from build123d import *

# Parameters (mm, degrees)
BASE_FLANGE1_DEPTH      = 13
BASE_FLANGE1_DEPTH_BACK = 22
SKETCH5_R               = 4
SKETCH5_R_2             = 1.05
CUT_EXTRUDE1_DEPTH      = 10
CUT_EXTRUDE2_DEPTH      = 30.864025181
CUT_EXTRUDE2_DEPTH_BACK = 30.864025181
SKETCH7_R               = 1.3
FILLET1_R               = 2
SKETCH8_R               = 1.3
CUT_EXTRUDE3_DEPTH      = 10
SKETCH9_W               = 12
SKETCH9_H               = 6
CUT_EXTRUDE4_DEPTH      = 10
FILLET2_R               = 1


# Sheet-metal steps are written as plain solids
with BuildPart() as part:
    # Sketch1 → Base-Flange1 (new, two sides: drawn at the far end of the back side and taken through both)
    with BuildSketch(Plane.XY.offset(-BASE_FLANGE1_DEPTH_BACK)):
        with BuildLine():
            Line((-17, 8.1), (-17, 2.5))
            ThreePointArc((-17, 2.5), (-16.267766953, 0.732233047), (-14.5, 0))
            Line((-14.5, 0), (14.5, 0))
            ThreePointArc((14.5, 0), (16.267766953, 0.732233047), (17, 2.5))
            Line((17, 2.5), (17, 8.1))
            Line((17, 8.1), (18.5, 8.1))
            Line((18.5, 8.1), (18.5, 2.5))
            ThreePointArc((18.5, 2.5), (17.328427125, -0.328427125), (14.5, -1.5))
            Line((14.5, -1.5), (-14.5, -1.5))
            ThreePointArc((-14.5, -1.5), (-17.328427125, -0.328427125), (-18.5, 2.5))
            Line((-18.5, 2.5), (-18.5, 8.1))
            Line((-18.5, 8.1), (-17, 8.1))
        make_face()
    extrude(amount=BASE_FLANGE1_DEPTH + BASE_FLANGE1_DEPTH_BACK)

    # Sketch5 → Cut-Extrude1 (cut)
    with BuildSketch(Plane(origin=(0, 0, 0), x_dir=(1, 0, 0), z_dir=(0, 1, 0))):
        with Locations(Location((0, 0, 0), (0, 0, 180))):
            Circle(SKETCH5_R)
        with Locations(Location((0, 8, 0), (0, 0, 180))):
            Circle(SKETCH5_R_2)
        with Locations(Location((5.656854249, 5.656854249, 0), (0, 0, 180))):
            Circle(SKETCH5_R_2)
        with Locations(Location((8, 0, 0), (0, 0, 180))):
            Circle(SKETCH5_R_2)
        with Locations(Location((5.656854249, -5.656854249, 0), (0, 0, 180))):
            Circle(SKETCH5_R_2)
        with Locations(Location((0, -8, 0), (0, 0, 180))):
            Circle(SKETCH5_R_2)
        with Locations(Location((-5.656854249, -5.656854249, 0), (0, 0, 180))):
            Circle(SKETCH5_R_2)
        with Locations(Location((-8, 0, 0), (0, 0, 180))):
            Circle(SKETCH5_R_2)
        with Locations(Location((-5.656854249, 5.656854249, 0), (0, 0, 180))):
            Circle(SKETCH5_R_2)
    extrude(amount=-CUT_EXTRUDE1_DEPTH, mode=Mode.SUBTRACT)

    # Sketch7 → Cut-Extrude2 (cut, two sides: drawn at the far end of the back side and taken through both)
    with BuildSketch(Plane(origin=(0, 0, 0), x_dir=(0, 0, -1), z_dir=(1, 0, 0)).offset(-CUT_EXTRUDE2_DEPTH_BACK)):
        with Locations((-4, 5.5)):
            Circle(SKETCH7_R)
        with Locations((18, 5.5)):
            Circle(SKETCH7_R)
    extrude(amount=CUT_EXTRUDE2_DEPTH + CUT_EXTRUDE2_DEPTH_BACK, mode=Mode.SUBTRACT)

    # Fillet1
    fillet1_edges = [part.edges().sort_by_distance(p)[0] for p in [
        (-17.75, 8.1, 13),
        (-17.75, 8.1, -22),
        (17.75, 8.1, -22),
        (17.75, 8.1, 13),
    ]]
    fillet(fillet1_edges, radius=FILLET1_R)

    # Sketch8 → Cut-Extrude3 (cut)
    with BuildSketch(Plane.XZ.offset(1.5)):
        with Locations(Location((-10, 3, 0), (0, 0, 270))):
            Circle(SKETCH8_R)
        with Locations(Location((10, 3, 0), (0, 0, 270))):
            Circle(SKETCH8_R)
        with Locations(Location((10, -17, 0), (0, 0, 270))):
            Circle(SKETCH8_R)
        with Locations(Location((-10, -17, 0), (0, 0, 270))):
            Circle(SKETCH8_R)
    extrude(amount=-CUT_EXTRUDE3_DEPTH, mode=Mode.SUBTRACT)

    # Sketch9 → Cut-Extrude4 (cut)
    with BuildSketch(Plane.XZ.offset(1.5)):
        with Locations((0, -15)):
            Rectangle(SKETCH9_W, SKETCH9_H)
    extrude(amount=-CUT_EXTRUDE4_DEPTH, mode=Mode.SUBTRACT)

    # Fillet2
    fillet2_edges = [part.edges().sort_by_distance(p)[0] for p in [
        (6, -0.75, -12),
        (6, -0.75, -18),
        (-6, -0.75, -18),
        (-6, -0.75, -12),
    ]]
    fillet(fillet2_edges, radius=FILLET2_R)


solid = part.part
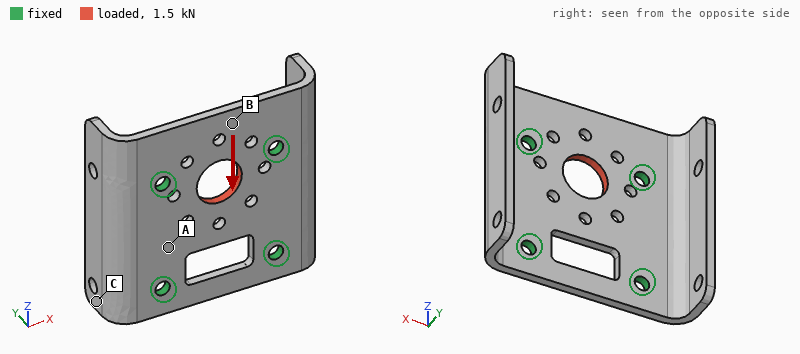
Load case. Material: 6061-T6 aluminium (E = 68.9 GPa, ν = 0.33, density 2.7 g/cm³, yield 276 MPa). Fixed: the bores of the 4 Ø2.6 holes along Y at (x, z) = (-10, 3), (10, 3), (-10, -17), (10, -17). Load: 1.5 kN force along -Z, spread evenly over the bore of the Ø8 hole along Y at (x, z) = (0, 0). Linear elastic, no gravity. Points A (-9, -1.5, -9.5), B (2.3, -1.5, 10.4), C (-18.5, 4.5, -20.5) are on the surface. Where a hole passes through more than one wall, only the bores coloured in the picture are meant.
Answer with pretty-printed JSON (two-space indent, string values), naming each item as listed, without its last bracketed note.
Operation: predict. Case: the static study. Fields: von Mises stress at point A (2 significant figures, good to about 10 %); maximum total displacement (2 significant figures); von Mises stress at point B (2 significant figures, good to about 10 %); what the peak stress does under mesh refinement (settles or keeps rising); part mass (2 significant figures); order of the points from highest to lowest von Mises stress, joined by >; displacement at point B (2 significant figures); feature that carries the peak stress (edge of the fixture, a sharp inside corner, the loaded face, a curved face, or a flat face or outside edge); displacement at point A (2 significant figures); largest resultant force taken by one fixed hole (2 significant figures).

{
  "von Mises stress at point A": "17 MPa",
  "maximum total displacement": "11 µm",
  "von Mises stress at point B": "31 MPa",
  "what the peak stress does under mesh refinement": "keeps rising",
  "part mass": "6.4 g",
  "order of the points from highest to lowest von Mises stress, joined by >": "B > A > C",
  "displacement at point B": "8.0 µm",
  "feature that carries the peak stress": "edge of the fixture",
  "displacement at point A": "2.3 µm",
  "largest resultant force taken by one fixed hole": "540 N"
}
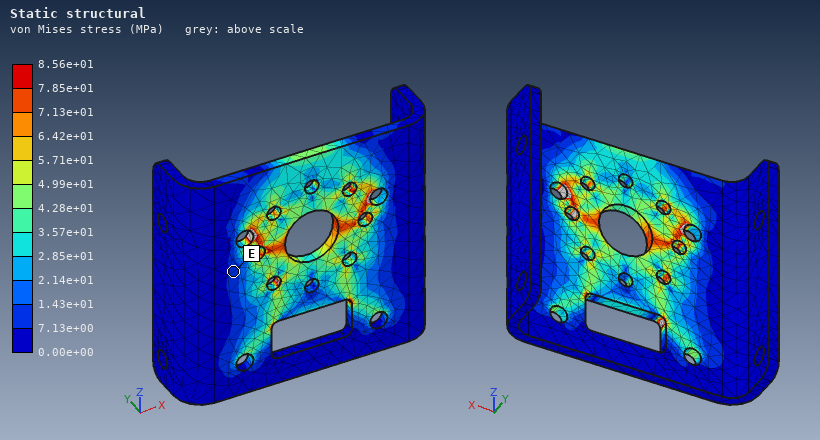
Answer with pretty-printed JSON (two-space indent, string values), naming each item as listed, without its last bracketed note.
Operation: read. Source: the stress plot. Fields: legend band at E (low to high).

{
  "legend band at E": "7.13e+00 to 1.43e+01 MPa"
}
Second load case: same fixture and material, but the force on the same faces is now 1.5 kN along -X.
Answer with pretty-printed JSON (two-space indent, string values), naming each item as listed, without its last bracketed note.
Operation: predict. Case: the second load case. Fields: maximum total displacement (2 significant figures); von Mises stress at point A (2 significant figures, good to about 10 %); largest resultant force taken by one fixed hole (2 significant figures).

{
  "maximum total displacement": "8.0 µm",
  "von Mises stress at point A": "11 MPa",
  "largest resultant force taken by one fixed hole": "610 N"
}
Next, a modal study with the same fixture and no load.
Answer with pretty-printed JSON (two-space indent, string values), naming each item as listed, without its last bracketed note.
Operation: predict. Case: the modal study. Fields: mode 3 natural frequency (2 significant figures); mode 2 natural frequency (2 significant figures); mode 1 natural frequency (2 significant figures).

{
  "mode 3 natural frequency": "8600 Hz",
  "mode 2 natural frequency": "6400 Hz",
  "mode 1 natural frequency": "6300 Hz"
}
